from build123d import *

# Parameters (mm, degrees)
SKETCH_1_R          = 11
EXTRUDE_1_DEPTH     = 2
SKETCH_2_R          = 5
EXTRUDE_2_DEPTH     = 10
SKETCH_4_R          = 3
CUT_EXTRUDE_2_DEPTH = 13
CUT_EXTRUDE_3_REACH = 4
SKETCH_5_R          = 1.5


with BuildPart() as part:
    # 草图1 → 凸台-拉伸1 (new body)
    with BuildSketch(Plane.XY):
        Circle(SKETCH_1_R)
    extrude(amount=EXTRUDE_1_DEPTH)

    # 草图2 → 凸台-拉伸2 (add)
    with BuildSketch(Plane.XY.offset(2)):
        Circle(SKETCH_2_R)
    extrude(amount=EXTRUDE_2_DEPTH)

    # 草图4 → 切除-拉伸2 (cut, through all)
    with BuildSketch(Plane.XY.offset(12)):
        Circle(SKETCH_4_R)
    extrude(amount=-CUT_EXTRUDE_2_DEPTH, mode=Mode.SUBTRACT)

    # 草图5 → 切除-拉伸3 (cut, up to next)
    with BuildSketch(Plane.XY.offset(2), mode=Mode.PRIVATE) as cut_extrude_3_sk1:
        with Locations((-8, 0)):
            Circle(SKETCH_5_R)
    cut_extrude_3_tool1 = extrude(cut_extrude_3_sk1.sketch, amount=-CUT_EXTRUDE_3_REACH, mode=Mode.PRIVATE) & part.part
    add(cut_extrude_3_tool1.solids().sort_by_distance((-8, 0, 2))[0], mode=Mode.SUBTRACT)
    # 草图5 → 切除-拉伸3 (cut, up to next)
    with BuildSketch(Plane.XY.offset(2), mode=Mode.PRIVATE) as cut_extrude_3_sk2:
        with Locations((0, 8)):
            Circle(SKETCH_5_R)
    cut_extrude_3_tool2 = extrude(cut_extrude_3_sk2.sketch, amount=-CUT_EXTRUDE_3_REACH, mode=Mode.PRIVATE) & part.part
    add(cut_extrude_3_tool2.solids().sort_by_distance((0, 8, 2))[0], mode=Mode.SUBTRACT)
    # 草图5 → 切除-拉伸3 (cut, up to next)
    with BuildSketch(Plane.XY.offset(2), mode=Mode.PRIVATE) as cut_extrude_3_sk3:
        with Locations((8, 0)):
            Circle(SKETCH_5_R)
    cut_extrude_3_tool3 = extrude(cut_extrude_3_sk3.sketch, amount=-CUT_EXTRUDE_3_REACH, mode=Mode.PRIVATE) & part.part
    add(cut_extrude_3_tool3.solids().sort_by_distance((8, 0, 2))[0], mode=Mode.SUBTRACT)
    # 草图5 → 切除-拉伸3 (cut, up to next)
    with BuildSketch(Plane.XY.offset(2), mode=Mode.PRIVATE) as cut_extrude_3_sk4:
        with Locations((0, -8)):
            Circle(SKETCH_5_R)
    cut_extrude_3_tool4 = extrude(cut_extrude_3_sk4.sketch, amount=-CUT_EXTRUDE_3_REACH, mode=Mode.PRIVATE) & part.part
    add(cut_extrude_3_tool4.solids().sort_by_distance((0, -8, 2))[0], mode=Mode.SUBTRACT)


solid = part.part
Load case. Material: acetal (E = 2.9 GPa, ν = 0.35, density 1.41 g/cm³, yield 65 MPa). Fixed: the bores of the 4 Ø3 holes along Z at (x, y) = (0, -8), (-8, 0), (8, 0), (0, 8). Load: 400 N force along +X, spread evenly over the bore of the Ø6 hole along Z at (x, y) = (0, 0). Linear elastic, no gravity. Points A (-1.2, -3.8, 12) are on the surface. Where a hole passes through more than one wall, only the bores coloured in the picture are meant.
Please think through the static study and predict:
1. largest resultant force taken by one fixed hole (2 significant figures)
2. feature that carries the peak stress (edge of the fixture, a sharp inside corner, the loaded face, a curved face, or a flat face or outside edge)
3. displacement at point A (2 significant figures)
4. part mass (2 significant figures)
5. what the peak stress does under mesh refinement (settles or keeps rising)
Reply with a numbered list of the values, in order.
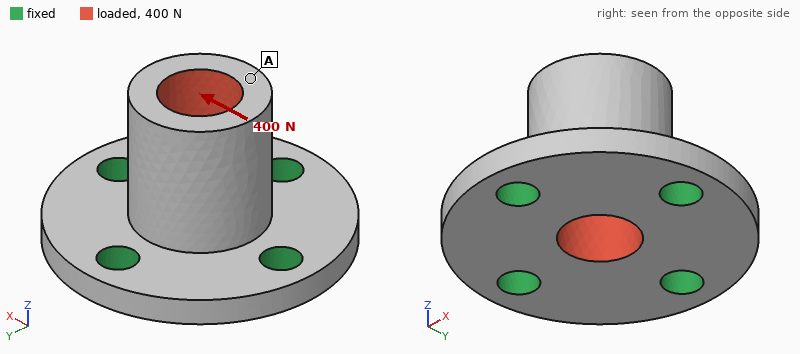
1. 200 N
2. edge of the fixture
3. 0.20 mm
4. 1.6 g
5. keeps rising
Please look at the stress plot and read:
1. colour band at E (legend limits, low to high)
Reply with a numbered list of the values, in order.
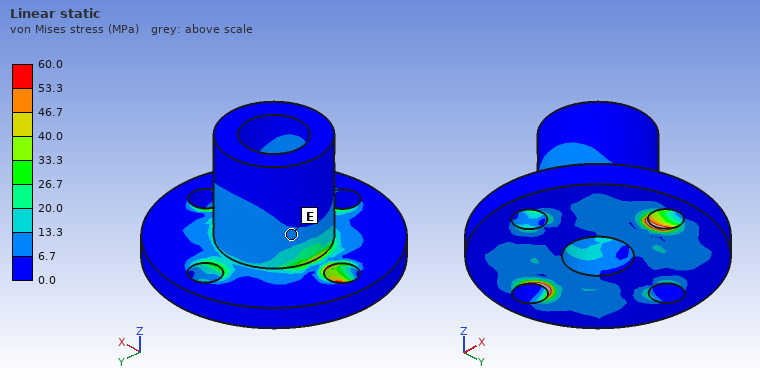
1. 6.7 to 13.3 MPa
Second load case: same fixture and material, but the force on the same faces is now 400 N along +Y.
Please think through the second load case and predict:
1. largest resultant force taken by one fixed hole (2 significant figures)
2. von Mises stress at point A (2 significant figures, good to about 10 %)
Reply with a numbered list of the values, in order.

1. 200 N
2. 5.0 MPa
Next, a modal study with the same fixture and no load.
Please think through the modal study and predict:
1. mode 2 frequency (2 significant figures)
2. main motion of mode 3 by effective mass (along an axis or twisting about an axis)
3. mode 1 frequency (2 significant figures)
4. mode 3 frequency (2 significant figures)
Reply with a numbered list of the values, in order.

1. 8700 Hz
2. along Z
3. 8700 Hz
4. 15 kHz
